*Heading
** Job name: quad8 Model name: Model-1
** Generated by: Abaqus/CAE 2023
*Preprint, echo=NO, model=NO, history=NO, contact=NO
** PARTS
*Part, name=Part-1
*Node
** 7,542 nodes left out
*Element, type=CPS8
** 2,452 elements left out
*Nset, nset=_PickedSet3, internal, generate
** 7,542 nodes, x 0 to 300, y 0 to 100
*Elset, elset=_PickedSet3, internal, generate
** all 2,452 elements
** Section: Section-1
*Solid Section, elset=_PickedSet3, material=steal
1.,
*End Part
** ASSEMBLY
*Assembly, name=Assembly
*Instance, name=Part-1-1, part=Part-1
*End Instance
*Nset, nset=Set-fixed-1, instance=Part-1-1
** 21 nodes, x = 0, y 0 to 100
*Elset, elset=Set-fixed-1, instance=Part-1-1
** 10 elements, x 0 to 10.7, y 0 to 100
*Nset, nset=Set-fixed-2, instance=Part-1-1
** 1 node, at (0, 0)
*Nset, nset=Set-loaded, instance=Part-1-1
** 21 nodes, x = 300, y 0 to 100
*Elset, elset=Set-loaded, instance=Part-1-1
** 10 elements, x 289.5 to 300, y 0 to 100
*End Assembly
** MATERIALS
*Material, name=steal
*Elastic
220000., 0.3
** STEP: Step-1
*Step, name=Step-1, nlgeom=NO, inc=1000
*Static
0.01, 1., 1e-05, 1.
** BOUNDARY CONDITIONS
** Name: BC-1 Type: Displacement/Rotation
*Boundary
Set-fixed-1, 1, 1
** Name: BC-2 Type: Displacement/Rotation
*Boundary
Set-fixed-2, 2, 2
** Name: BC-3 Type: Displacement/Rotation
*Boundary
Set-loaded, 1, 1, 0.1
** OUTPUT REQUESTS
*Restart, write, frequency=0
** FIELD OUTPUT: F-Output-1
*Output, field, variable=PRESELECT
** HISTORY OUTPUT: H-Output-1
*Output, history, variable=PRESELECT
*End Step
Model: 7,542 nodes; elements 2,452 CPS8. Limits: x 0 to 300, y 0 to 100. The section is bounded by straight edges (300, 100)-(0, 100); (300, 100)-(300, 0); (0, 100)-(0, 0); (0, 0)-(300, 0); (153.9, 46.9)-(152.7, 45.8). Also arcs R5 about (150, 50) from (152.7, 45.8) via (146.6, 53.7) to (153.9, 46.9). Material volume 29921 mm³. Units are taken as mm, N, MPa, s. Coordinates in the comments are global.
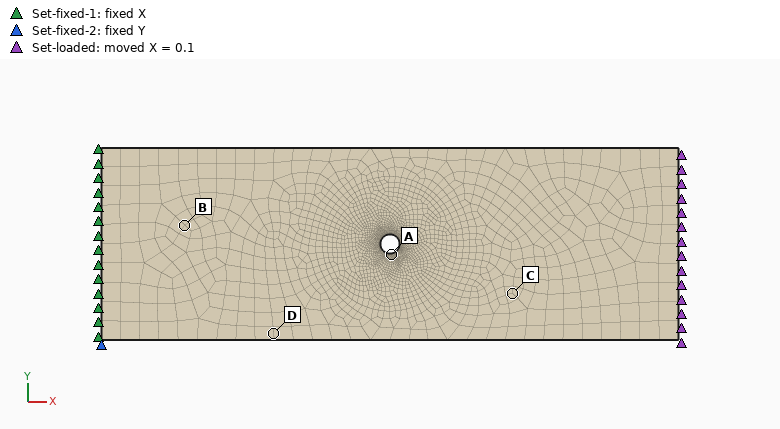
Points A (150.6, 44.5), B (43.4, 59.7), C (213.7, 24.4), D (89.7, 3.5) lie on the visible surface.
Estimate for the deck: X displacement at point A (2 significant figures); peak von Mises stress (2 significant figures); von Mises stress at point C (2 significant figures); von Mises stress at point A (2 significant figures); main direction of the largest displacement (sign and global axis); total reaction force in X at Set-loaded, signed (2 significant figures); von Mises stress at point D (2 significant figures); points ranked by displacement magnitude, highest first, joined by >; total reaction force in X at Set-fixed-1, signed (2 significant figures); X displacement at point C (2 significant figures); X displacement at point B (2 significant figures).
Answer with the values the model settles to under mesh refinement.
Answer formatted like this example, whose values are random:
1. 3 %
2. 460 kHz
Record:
1. 0.051 mm
2. 220 MPa
3. 73 MPa
4. 170 MPa
5. +X
6. 7300 N
7. 74 MPa
8. C > A > D > B
9. -7300 N
10. 0.071 mm
11. 0.014 mm
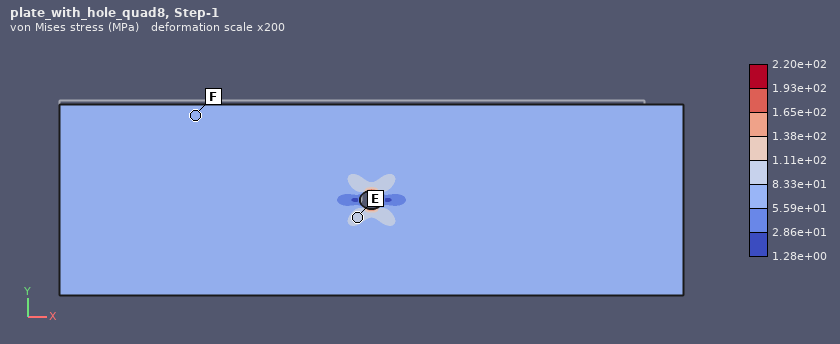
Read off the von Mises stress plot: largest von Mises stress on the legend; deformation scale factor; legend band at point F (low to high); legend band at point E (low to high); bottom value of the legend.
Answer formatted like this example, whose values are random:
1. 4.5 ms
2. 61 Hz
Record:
1. 2.20e+02 MPa
2. 200
3. 5.59e+01 to 8.33e+01 MPa
4. 8.33e+01 to 1.11e+02 MPa
5. 1.28e+00 MPa
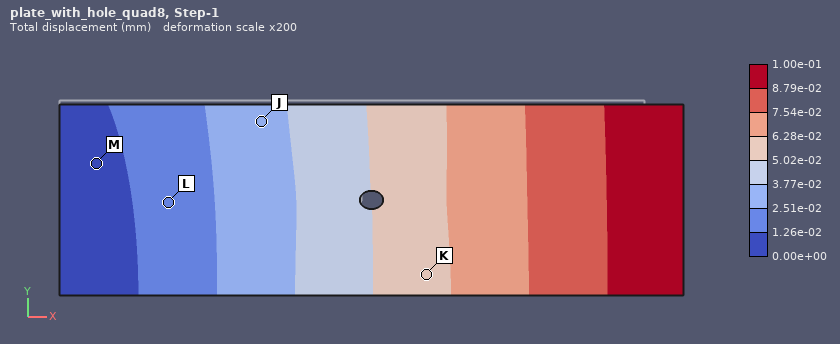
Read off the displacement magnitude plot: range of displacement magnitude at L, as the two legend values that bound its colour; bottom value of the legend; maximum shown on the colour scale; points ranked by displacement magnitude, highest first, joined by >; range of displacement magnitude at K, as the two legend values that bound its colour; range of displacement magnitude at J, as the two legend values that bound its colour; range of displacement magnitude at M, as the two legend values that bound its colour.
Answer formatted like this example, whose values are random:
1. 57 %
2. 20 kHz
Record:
1. 1.26e-02 to 2.51e-02 mm
2. 0.00e+00 mm
3. 1.00e-01 mm
4. K > J > L > M
5. 5.02e-02 to 6.28e-02 mm
6. 2.51e-02 to 3.77e-02 mm
7. 0.00e+00 to 1.26e-02 mm
